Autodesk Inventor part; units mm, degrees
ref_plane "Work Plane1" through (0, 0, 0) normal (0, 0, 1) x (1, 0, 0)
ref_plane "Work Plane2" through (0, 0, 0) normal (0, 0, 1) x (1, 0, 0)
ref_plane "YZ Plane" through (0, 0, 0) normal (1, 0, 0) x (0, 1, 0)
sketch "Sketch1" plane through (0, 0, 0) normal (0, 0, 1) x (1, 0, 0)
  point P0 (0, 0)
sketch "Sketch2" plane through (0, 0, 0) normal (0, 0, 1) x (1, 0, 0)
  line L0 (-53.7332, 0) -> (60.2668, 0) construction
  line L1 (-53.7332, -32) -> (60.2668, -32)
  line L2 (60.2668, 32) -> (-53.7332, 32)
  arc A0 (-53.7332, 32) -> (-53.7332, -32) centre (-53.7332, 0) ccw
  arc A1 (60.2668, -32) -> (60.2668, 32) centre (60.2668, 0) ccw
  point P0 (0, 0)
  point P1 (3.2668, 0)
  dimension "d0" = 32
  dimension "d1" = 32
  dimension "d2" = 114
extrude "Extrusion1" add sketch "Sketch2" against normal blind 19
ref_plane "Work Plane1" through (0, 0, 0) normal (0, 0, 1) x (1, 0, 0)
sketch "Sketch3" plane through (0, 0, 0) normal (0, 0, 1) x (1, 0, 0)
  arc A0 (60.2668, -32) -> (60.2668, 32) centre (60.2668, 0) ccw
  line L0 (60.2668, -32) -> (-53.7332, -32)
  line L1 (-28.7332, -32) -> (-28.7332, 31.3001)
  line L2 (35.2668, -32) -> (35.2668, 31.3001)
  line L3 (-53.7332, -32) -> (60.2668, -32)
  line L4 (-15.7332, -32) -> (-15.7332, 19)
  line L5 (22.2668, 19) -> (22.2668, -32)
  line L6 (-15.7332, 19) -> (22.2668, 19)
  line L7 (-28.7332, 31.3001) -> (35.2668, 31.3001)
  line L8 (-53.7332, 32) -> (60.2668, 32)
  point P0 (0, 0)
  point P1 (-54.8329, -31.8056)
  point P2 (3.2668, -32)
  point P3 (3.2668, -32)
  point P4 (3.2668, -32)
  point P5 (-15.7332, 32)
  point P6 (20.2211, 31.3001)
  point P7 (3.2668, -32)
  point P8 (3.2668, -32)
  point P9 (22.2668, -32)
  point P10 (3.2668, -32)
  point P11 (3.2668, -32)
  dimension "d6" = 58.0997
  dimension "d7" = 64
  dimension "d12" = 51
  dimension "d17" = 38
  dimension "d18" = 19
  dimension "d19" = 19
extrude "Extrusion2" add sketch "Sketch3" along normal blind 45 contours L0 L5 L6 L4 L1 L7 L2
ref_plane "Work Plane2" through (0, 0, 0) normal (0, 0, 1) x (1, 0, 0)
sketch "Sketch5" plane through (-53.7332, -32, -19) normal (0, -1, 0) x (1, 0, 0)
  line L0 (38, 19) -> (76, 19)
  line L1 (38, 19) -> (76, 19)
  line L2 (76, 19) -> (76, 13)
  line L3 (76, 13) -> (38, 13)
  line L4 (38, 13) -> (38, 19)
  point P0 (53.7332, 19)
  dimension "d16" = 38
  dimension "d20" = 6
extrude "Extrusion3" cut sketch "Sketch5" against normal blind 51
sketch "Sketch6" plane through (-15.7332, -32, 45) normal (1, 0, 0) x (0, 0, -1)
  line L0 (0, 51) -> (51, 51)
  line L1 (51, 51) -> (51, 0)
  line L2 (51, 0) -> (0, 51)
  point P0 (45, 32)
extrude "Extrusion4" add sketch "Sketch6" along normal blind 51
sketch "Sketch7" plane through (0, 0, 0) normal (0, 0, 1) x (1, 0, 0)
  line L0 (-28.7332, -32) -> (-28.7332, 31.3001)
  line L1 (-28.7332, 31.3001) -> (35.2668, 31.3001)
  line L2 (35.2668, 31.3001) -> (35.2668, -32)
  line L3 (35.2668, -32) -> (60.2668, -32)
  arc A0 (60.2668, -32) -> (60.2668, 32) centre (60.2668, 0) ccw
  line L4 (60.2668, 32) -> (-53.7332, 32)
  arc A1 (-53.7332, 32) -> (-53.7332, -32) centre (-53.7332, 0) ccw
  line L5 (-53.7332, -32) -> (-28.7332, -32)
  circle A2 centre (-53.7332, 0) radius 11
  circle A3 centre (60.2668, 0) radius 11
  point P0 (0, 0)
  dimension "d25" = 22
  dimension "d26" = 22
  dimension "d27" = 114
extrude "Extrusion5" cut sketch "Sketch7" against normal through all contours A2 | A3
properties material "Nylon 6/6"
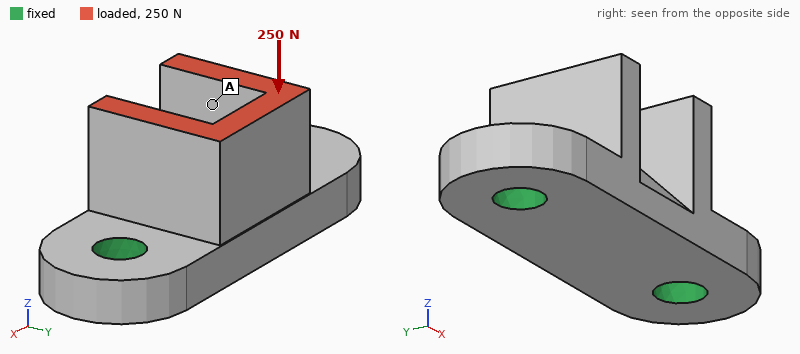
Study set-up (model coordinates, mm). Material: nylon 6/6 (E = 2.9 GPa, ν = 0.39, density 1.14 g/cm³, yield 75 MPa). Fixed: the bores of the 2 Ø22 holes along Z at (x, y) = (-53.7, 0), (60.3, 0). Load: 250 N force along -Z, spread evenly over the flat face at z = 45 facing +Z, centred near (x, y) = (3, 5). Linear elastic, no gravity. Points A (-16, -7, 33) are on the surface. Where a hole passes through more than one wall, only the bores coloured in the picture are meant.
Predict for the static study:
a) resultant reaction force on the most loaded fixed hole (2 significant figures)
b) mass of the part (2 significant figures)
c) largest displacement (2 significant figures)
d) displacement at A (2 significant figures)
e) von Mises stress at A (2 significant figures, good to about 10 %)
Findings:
130 N
360 g
12 µm
7.2 µm
0.12 MPa
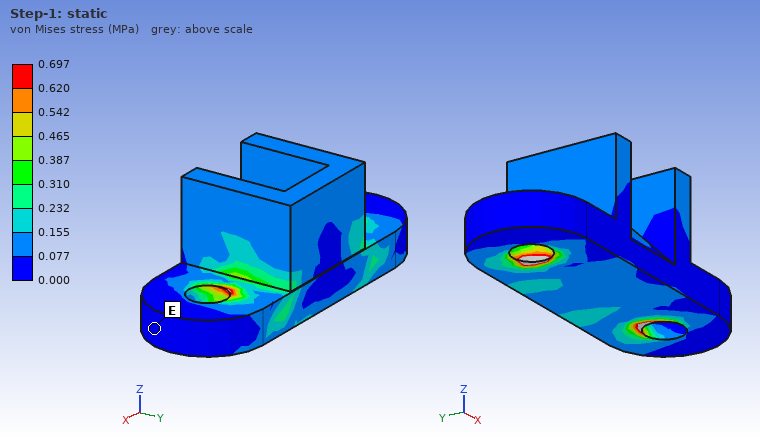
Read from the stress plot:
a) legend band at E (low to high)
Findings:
0.000 to 0.077 MPa
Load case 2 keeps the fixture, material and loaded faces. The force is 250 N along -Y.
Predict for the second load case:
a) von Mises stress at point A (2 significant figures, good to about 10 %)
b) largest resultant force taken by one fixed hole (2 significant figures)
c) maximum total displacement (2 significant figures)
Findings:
0.31 MPa
130 N
72 µm
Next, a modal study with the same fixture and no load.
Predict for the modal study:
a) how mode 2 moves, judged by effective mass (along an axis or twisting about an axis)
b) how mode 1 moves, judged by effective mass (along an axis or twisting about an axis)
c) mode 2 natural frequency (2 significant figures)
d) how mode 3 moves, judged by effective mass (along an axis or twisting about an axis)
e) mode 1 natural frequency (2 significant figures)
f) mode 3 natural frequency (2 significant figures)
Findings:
along Z
along Y
2000 Hz
along X
1100 Hz
2200 Hz
